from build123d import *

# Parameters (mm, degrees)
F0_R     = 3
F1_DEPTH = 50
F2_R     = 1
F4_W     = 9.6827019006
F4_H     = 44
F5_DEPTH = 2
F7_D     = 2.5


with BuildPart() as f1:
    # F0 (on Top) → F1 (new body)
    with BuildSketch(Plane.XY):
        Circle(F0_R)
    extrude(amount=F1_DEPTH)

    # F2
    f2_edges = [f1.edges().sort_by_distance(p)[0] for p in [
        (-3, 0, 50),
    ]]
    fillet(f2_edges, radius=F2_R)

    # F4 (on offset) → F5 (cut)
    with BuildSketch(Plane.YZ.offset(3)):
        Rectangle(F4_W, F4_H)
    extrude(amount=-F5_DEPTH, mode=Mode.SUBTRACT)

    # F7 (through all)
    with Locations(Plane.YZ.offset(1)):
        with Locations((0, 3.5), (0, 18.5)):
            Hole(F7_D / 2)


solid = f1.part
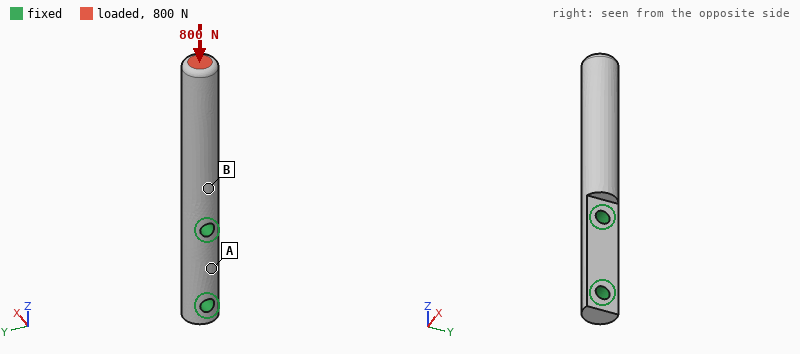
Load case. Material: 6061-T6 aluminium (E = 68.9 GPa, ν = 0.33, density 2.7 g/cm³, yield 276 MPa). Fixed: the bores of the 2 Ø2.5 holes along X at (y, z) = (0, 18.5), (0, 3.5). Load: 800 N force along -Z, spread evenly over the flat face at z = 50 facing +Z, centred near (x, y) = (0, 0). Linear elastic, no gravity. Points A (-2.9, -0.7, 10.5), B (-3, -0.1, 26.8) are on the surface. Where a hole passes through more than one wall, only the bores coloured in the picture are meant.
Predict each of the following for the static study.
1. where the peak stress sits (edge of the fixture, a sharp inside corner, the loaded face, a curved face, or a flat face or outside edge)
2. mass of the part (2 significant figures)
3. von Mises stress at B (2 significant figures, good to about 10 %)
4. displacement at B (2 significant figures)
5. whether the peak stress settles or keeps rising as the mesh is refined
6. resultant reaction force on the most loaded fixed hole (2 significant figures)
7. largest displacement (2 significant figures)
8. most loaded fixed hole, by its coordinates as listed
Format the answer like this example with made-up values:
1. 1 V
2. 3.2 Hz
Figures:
1. edge of the fixture
2. 3.2 g
3. 26 MPa
4. 9.0 µm
5. keeps rising
6. 780 N
7. 50 µm
8. (0, 18.5)
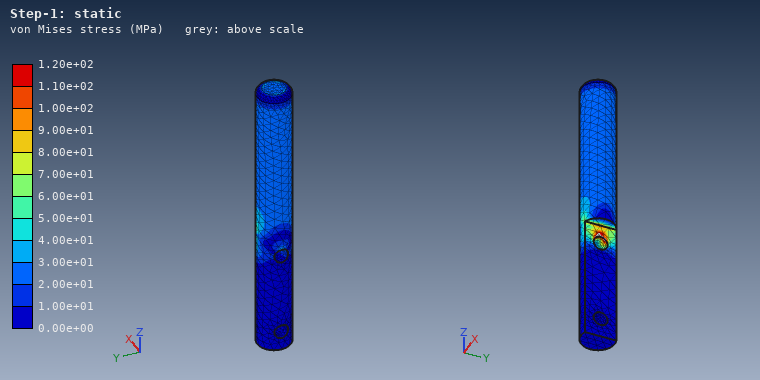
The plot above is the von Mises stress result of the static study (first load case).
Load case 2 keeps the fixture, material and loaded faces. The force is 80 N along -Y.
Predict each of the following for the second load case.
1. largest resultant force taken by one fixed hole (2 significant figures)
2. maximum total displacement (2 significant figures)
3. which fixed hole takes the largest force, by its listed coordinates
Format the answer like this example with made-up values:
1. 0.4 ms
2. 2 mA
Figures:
1. 120 N
2. 0.23 mm
3. (0, 18.5)
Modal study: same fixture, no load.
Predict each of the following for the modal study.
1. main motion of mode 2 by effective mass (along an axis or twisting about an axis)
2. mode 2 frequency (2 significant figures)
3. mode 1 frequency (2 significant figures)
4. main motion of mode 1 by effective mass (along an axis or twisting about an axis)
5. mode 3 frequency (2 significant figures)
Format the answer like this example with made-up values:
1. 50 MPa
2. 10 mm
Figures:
1. along Y
2. 3800 Hz
3. 3300 Hz
4. along X
5. 22 kHz
